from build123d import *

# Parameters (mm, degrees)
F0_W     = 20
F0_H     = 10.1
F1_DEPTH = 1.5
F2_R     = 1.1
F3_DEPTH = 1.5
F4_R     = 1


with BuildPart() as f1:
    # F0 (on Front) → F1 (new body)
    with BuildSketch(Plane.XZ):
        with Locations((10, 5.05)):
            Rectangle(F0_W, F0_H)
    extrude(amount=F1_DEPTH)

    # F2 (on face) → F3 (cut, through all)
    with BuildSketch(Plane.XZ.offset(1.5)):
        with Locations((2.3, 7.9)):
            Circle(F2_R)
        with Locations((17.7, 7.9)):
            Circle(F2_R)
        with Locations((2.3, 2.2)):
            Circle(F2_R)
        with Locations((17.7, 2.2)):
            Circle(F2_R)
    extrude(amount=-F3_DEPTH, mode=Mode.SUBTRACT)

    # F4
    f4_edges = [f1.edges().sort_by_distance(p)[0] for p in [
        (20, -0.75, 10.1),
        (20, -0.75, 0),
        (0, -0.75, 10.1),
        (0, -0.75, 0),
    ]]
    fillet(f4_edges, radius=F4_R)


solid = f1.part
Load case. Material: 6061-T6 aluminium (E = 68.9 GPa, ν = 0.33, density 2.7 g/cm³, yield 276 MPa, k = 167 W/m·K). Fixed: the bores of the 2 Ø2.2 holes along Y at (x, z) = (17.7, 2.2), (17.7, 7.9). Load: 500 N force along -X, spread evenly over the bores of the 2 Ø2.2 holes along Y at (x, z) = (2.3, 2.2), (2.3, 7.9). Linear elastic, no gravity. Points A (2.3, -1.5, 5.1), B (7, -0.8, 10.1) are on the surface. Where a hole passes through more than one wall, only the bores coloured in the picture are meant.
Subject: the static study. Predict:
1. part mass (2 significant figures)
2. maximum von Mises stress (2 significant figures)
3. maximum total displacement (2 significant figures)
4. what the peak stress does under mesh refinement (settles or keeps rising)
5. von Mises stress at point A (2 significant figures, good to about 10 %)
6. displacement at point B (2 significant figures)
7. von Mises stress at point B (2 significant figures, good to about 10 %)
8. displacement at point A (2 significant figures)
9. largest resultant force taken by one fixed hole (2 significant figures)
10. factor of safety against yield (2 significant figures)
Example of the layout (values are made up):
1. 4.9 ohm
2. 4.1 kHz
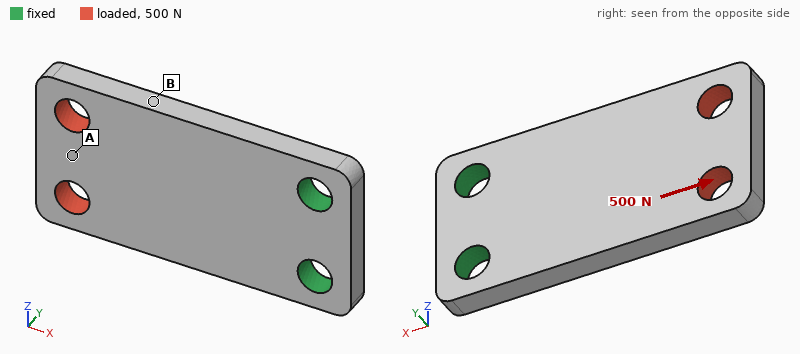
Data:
1. 0.75 g
2. 93 MPa
3. 9.3 µm
4. settles
5. 14 MPa
6. 5.1 µm
7. 36 MPa
8. 6.9 µm
9. 250 N
10. 3.0
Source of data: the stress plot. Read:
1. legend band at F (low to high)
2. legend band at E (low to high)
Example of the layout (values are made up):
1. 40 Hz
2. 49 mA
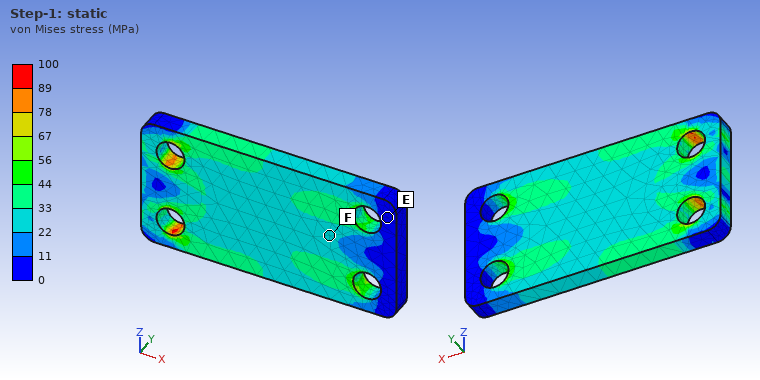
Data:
1. 22 to 33 MPa
2. 0 to 11 MPa
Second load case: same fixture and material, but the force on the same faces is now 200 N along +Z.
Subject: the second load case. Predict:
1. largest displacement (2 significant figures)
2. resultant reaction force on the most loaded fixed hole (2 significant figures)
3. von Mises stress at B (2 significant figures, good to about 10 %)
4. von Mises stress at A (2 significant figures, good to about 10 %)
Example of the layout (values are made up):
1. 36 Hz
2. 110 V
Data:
1. 44 µm
2. 440 N
3. 37 MPa
4. 28 MPa
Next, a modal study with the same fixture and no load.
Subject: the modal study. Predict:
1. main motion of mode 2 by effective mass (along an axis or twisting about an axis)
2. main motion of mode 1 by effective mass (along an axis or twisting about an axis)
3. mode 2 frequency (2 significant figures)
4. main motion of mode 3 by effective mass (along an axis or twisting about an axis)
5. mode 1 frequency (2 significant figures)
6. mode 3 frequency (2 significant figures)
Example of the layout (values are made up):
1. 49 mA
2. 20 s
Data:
1. twisting about X
2. along Y
3. 16 kHz
4. along Z
5. 4600 Hz
6. 23 kHz
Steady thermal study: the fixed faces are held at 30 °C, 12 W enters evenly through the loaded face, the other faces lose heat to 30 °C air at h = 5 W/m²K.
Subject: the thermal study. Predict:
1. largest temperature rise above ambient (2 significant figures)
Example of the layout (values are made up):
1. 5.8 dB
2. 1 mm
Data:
1. 77 K
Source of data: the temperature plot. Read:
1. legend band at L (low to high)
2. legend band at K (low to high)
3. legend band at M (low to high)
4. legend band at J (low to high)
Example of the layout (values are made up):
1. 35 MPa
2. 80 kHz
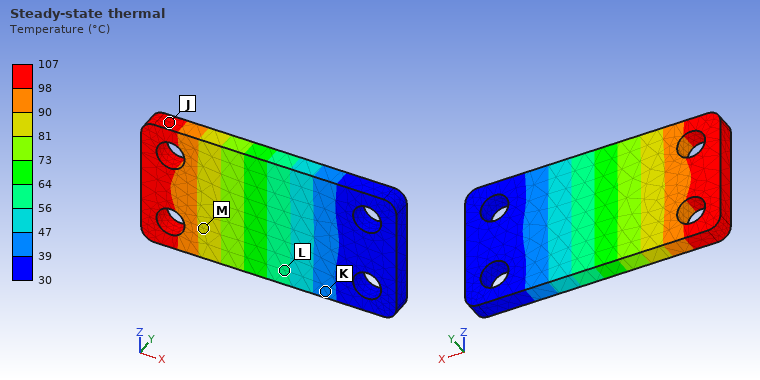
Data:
1. 56 to 64 °C
2. 39 to 47 °C
3. 81 to 90 °C
4. 98 to 107 °C
